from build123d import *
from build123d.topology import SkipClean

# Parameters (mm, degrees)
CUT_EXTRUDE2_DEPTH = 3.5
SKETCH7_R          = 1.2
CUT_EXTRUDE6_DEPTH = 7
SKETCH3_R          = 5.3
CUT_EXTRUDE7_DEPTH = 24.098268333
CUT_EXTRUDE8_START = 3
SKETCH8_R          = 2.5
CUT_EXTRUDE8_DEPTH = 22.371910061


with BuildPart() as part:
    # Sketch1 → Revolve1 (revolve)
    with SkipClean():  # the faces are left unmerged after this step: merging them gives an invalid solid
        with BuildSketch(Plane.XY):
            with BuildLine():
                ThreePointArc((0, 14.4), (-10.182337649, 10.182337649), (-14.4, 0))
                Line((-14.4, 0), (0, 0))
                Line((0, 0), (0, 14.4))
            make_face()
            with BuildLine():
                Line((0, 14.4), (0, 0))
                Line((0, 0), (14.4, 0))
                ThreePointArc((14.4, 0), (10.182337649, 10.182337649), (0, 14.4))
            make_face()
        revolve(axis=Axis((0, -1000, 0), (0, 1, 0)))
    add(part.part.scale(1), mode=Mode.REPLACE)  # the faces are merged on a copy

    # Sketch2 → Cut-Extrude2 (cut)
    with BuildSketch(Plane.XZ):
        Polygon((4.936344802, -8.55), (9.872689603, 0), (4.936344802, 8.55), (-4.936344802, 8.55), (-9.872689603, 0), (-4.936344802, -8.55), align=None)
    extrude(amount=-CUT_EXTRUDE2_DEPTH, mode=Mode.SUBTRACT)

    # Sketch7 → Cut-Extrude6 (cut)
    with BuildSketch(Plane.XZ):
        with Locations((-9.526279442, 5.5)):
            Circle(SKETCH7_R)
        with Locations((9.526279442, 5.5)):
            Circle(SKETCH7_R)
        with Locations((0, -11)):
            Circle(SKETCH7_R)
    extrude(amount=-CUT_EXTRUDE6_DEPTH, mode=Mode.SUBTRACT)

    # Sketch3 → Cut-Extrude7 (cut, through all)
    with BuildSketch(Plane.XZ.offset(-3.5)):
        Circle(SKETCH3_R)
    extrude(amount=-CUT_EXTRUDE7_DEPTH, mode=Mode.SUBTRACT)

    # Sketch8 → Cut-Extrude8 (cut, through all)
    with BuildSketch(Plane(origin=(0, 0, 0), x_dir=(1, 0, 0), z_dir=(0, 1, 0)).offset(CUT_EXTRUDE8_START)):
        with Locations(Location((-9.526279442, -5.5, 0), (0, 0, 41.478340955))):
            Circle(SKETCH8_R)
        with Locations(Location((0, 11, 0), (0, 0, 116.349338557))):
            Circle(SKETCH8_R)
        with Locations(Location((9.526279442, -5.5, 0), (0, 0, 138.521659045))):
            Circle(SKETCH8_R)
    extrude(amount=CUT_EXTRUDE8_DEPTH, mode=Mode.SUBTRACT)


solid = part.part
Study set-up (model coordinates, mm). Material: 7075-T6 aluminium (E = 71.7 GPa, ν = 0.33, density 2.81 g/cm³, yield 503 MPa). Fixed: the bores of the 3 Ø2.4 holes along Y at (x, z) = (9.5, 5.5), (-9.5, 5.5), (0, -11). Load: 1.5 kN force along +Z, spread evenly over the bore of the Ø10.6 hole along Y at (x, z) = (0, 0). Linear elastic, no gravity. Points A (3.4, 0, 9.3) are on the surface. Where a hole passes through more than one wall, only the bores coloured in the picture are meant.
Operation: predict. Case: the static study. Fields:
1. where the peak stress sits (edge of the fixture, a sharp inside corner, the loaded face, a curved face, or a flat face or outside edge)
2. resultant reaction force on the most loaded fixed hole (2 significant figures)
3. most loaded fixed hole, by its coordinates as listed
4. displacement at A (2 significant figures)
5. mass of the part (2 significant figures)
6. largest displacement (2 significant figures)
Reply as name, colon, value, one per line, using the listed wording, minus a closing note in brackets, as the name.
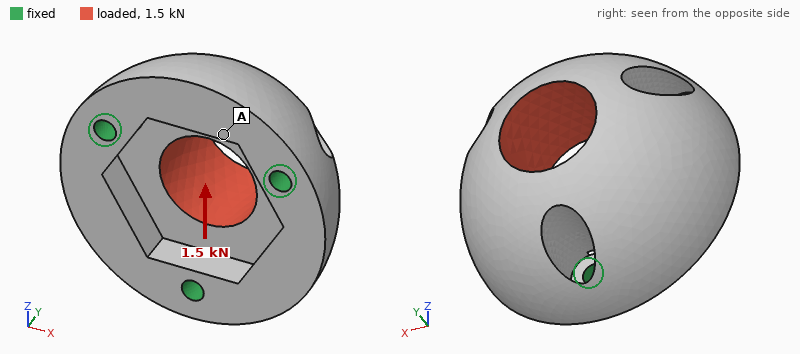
where the peak stress sits: a flat face or outside edge
resultant reaction force on the most loaded fixed hole: 750 N
most loaded fixed hole, by its coordinates as listed: (0, -11)
displacement at A: 3.5 µm
mass of the part: 11 g
largest displacement: 11 µm
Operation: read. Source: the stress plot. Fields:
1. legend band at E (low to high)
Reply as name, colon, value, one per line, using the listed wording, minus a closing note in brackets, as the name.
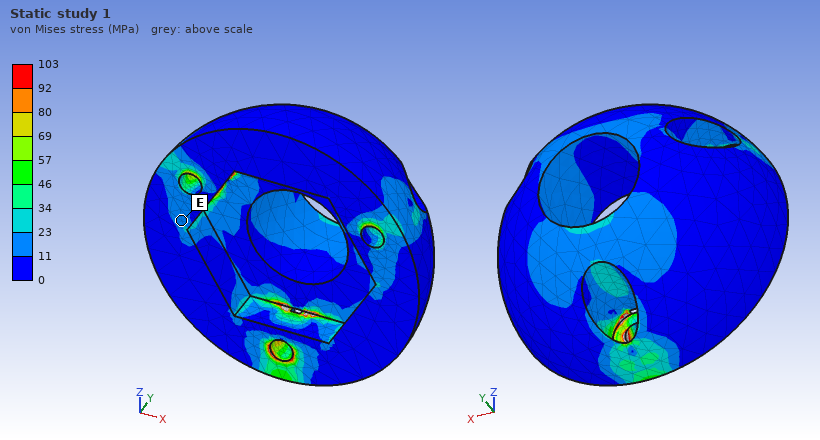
legend band at E: 11 to 23 MPa
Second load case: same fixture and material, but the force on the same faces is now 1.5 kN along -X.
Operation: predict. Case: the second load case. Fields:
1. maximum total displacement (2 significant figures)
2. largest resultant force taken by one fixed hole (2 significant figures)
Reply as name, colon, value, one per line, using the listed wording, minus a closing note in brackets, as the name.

maximum total displacement: 10 µm
largest resultant force taken by one fixed hole: 690 N
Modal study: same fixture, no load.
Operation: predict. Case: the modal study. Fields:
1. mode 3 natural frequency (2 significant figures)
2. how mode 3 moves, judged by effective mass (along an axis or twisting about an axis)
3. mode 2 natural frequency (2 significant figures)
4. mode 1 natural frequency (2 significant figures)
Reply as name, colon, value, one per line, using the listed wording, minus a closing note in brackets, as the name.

mode 3 natural frequency: 33 kHz
how mode 3 moves, judged by effective mass: along Y
mode 2 natural frequency: 25 kHz
mode 1 natural frequency: 25 kHz
